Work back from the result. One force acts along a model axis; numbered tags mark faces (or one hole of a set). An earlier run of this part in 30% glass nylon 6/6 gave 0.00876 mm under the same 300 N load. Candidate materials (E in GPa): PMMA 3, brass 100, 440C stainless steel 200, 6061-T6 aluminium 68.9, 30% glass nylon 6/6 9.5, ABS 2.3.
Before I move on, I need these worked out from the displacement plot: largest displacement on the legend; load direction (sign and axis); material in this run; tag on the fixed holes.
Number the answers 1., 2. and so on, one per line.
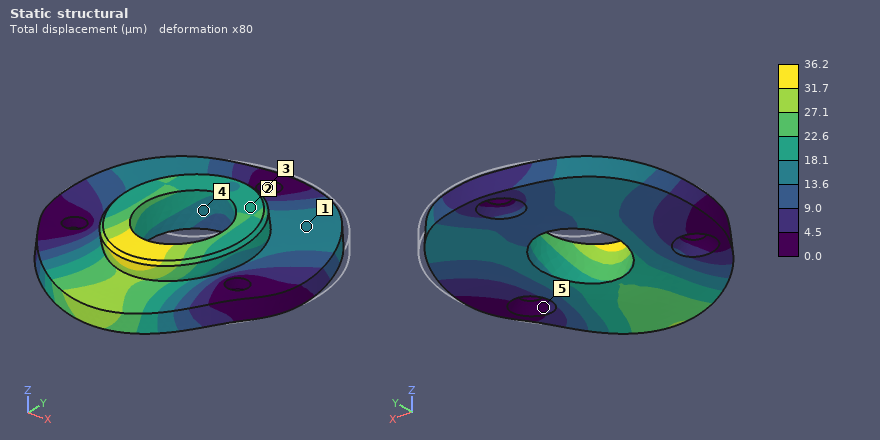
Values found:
1. 36.2 µm
2. -Y
3. ABS
4. 3
